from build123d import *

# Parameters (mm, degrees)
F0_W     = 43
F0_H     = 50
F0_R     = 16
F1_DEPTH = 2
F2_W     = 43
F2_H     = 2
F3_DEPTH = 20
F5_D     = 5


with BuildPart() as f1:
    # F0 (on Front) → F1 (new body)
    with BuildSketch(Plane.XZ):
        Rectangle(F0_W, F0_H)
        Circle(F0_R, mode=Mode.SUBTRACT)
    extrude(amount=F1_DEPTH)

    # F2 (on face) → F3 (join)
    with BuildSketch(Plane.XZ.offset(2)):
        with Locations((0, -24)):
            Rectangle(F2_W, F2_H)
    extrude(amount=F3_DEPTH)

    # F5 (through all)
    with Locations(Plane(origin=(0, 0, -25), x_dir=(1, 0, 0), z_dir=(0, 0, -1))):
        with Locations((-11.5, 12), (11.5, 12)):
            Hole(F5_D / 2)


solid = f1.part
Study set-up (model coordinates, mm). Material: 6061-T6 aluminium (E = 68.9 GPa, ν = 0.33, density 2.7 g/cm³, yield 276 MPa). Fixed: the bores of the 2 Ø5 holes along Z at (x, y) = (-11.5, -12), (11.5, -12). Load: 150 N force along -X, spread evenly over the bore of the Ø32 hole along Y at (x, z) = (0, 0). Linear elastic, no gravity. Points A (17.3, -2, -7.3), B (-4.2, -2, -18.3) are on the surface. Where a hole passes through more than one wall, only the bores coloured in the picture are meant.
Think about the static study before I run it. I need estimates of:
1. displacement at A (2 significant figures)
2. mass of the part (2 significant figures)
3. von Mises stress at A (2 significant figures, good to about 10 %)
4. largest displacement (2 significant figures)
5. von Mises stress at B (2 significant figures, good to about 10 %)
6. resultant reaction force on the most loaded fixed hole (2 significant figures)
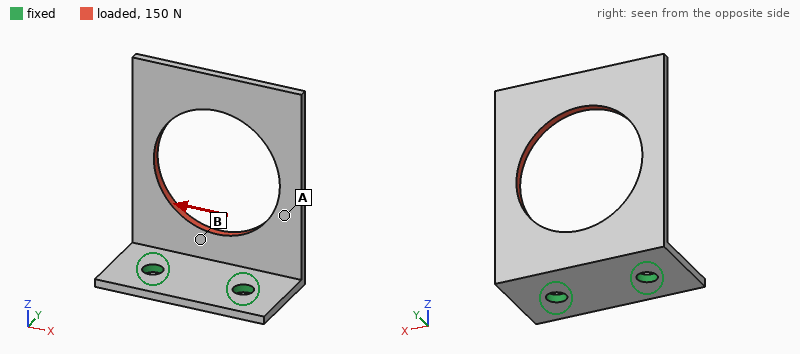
0.081 mm
12 g
15 MPa
0.18 mm
32 MPa
160 N
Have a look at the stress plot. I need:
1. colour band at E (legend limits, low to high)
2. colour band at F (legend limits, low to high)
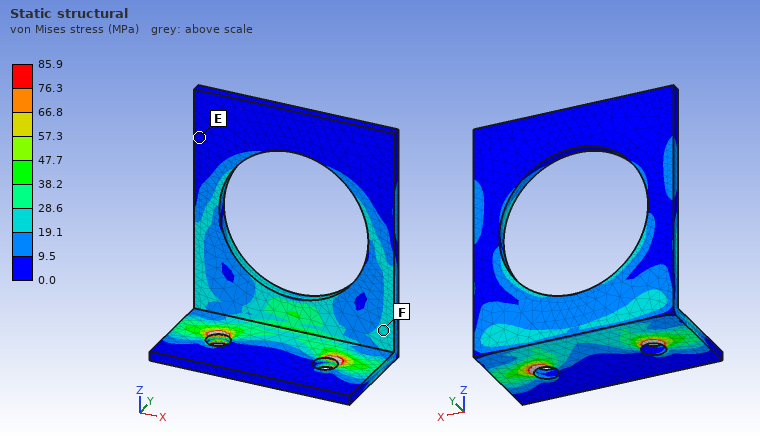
0.0 to 9.5 MPa
19.1 to 28.6 MPa
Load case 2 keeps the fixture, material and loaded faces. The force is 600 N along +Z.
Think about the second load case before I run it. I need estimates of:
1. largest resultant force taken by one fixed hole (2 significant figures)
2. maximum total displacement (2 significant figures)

300 N
0.73 mm
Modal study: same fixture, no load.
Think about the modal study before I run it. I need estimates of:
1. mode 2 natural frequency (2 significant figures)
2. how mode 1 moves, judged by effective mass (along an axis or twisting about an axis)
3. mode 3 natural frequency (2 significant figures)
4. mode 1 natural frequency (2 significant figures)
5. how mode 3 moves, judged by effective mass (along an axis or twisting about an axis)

1300 Hz
along Y
2100 Hz
470 Hz
along X
